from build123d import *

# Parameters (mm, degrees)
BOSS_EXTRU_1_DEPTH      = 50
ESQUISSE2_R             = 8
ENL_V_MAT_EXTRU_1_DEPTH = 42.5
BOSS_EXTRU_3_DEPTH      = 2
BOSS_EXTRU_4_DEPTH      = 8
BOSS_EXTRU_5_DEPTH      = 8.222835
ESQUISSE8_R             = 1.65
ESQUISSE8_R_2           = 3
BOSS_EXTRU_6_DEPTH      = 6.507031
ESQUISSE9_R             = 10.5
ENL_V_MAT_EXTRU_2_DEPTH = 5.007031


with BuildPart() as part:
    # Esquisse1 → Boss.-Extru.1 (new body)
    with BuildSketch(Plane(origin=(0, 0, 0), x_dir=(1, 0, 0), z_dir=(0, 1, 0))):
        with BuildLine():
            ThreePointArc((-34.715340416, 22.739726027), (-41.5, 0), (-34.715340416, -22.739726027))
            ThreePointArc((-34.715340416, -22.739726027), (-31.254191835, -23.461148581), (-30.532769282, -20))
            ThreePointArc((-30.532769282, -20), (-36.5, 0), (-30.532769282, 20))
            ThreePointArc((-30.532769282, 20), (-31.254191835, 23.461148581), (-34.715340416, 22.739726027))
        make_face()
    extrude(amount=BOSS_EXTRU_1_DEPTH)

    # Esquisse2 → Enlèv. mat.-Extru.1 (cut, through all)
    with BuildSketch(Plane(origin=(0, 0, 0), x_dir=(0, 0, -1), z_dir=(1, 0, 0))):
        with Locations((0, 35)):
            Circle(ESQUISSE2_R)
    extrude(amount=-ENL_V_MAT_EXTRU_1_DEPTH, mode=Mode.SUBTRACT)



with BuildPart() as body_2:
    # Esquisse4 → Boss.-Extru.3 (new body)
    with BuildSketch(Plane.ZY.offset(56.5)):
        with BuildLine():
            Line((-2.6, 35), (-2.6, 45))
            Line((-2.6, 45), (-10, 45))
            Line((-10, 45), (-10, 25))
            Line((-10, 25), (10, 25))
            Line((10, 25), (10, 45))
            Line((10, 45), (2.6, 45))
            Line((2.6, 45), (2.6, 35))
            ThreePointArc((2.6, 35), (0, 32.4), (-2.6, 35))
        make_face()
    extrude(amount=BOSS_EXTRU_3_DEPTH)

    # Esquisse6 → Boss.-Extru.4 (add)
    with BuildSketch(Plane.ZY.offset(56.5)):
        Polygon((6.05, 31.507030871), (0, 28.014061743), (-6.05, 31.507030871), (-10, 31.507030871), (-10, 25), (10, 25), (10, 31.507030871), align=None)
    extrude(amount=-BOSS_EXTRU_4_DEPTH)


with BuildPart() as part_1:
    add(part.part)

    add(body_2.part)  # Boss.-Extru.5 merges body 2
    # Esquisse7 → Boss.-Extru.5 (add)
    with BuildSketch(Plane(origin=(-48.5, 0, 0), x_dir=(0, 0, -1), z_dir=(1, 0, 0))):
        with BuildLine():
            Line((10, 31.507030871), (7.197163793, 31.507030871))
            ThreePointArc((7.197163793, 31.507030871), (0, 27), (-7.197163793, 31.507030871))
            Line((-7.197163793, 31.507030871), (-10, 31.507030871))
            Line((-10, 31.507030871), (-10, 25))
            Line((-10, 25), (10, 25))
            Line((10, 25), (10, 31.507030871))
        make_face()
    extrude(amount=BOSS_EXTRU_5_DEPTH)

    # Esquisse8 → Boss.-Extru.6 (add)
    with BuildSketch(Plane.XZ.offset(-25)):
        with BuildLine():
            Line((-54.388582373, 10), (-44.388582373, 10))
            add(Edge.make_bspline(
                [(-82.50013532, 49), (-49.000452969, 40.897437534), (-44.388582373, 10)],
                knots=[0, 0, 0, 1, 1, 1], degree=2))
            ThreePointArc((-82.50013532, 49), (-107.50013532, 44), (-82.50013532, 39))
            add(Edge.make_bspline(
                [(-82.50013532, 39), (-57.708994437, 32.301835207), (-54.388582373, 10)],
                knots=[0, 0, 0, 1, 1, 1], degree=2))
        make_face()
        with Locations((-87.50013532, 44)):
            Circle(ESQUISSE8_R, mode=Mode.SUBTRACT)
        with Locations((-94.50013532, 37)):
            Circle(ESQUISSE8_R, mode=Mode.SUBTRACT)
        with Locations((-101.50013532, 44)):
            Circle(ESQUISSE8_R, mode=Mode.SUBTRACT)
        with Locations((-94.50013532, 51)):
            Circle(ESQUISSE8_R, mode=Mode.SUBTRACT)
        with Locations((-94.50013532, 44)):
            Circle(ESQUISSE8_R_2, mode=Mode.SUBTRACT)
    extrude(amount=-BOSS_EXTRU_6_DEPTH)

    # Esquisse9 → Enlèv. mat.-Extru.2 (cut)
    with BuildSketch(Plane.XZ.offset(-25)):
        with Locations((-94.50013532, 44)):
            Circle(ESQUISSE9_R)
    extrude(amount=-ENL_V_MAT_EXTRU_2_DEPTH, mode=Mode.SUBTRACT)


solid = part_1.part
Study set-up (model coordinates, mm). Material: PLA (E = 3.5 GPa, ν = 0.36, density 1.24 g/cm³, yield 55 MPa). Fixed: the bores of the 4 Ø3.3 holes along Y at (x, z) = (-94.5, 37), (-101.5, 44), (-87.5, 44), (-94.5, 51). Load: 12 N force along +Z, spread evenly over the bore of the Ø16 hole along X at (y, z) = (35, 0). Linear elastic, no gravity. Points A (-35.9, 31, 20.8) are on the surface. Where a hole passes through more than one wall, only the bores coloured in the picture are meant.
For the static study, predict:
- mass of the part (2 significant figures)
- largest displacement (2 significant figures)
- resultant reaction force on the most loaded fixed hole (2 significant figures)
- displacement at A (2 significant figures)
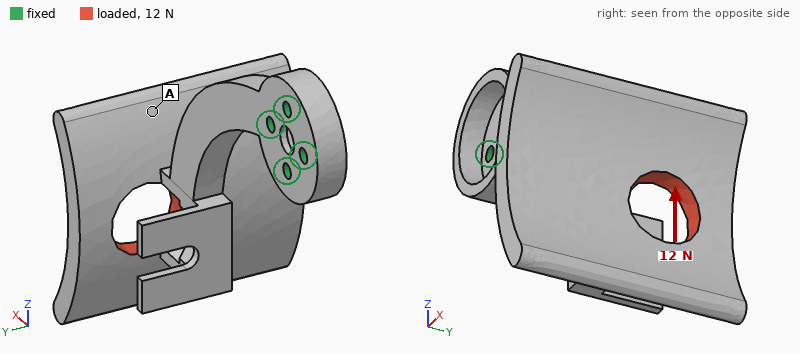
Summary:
23 g
1.2 mm
35 N
0.53 mm
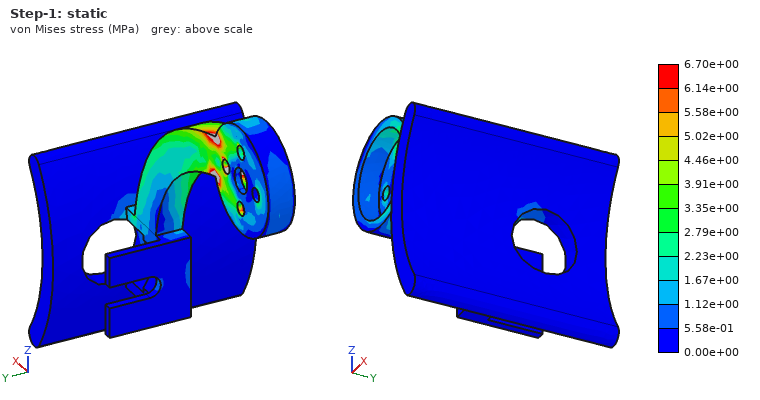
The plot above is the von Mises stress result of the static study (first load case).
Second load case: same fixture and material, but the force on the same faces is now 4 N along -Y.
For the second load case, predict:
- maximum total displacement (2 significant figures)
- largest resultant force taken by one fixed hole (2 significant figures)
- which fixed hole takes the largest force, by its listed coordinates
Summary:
1.4 mm
27 N
(-87.5, 44)
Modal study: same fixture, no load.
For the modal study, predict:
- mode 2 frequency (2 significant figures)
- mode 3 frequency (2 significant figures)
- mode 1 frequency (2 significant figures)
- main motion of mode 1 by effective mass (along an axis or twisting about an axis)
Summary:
130 Hz
220 Hz
75 Hz
along Y
